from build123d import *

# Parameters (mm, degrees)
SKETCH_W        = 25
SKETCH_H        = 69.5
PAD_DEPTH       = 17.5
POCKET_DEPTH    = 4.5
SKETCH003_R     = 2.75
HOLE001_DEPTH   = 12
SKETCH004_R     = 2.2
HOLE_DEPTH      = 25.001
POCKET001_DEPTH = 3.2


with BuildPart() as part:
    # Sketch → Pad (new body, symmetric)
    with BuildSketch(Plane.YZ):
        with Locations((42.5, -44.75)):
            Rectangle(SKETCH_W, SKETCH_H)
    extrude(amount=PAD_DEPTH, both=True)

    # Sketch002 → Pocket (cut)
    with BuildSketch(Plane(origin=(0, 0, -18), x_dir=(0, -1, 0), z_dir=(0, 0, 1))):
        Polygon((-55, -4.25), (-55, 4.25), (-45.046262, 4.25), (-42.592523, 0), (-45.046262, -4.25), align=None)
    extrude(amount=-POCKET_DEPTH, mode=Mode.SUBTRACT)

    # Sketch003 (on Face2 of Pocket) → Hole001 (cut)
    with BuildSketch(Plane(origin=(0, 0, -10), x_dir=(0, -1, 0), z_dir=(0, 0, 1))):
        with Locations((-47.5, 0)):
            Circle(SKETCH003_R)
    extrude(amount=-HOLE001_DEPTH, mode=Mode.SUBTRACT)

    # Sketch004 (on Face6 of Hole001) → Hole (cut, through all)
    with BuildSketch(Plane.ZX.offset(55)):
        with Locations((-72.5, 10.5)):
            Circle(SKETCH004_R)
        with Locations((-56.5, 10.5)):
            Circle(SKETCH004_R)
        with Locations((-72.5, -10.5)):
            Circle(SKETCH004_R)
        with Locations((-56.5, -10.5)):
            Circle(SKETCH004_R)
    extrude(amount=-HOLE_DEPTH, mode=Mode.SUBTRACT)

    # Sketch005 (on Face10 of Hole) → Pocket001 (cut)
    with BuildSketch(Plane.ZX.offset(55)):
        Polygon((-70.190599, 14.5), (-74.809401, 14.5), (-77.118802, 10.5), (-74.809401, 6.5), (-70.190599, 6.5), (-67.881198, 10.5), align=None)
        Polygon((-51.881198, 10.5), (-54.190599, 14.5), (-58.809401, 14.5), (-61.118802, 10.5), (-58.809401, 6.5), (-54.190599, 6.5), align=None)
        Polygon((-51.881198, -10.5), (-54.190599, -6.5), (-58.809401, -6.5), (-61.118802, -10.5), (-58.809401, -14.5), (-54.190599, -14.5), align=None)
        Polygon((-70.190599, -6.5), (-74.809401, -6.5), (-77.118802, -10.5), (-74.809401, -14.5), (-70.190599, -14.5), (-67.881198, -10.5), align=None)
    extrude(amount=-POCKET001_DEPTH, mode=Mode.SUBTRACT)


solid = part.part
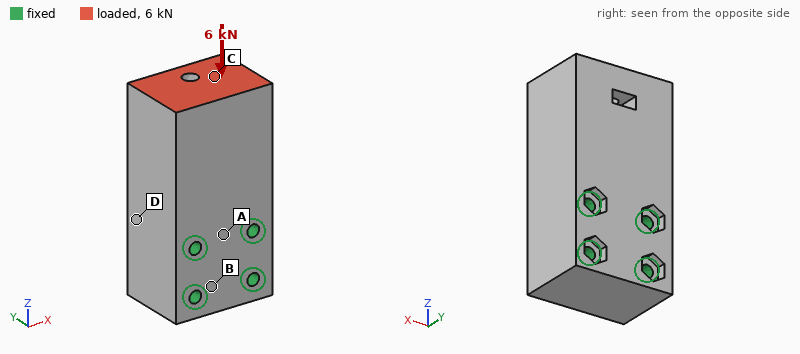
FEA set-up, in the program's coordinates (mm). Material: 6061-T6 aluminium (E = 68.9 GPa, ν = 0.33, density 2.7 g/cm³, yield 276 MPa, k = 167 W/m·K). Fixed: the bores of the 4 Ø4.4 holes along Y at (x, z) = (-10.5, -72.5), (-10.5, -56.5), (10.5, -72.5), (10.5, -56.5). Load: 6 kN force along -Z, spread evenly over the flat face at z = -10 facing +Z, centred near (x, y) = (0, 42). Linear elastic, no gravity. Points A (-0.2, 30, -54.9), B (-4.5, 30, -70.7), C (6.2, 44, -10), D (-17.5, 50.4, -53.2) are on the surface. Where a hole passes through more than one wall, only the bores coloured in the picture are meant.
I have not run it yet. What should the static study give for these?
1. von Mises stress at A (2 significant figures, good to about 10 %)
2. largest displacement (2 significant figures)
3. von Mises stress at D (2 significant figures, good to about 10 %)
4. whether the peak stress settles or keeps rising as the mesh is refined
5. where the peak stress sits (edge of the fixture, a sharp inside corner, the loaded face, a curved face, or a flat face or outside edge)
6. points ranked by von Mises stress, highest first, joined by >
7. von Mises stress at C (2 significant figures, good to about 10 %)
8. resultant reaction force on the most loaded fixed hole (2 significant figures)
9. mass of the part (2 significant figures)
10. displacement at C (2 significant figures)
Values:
2.7 MPa
6.5 µm
4.7 MPa
keeps rising
edge of the fixture
C > D > A > B
7.7 MPa
2.5 kN
160 g
5.3 µm
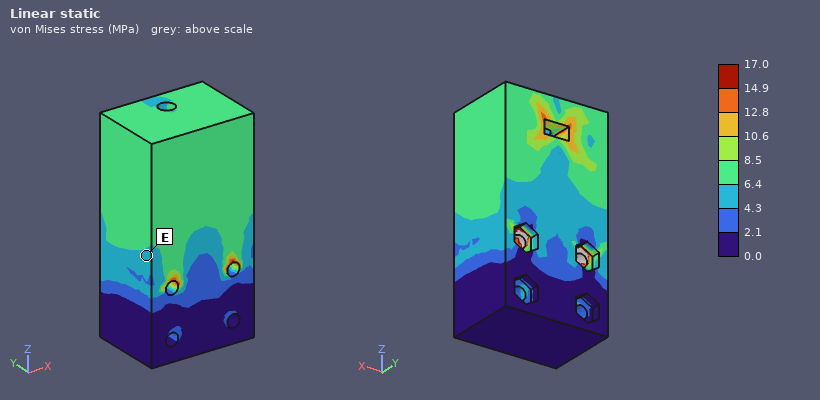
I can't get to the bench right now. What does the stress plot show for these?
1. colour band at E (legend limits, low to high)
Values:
4.3 to 6.4 MPa
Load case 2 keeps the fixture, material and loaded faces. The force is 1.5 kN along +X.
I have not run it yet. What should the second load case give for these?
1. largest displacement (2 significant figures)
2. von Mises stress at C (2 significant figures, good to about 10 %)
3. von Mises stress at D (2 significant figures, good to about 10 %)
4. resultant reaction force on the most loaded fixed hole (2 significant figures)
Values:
15 µm
4.0 MPa
9.2 MPa
2.6 kN
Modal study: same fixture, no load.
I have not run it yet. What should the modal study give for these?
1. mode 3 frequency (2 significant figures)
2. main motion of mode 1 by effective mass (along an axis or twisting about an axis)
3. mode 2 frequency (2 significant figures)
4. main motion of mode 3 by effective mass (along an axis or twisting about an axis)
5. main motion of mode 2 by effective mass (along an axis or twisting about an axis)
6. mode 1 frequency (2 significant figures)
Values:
15 kHz
along Y
9400 Hz
twisting about Z
along X
7200 Hz
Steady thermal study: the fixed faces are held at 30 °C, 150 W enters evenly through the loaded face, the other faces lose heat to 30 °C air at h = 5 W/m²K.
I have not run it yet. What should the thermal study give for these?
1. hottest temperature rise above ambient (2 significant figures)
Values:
51 K
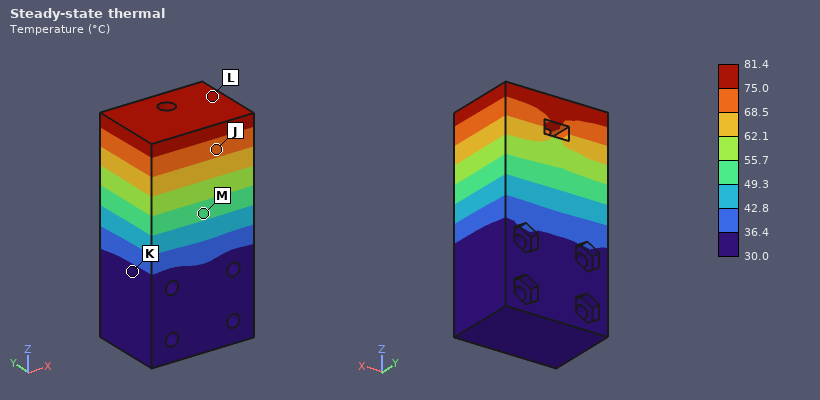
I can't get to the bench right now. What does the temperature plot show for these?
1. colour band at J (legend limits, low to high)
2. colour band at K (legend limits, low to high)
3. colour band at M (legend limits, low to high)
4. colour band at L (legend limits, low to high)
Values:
68.5 to 75.0 °C
30.0 to 36.4 °C
49.3 to 55.7 °C
75.0 to 81.4 °C
